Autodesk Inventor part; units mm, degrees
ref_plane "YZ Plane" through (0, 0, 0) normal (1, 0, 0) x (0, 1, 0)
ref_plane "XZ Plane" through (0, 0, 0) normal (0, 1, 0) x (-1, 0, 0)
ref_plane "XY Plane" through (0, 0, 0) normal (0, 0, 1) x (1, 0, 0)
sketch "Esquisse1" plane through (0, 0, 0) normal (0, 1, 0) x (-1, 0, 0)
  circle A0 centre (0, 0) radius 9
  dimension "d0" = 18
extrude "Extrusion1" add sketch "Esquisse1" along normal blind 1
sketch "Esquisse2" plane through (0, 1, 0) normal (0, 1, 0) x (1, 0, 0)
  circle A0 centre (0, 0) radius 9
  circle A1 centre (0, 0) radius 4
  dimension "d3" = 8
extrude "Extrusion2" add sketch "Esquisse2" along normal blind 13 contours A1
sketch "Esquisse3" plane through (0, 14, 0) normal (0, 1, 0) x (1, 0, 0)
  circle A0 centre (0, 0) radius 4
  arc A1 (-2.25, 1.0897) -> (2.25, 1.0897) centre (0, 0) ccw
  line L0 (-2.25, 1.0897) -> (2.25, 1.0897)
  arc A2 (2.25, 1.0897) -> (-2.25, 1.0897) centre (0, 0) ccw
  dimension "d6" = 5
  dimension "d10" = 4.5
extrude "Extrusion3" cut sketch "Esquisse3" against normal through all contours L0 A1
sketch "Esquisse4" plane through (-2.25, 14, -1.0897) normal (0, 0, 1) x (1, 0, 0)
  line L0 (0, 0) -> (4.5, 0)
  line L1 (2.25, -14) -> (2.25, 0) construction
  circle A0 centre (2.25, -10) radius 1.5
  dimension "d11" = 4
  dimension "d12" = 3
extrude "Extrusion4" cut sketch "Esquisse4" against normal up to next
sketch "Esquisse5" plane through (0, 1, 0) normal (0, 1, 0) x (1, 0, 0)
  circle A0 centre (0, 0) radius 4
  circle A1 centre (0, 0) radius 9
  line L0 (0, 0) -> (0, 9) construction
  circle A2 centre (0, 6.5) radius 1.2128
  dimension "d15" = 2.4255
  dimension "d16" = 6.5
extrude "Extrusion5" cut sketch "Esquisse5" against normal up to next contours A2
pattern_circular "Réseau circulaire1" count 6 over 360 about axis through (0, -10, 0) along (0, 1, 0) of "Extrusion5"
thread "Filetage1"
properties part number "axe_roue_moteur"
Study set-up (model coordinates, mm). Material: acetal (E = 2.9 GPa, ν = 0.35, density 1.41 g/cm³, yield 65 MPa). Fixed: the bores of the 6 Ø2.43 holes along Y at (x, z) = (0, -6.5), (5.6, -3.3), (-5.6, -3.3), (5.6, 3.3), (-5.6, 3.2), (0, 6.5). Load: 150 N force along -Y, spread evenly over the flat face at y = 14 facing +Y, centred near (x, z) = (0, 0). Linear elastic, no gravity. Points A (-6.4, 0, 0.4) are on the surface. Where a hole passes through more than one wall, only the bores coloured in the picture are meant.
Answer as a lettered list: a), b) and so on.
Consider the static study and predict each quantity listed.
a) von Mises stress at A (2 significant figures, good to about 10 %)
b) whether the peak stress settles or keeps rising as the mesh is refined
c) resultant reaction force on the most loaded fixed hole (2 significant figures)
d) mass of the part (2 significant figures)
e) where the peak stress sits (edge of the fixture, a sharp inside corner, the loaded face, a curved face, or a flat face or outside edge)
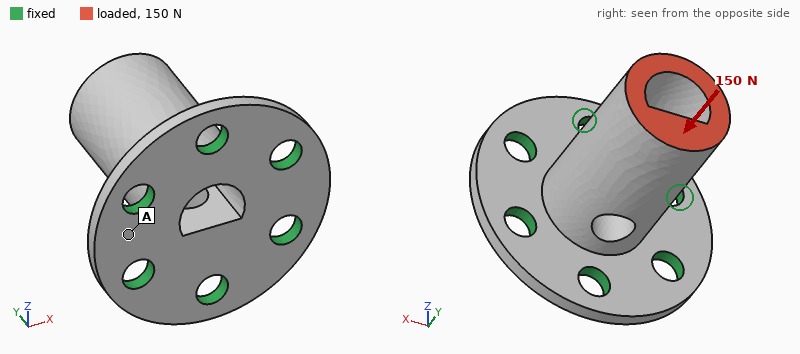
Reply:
a) 6.3 MPa
b) keeps rising
c) 30 N
d) 0.91 g
e) edge of the fixture
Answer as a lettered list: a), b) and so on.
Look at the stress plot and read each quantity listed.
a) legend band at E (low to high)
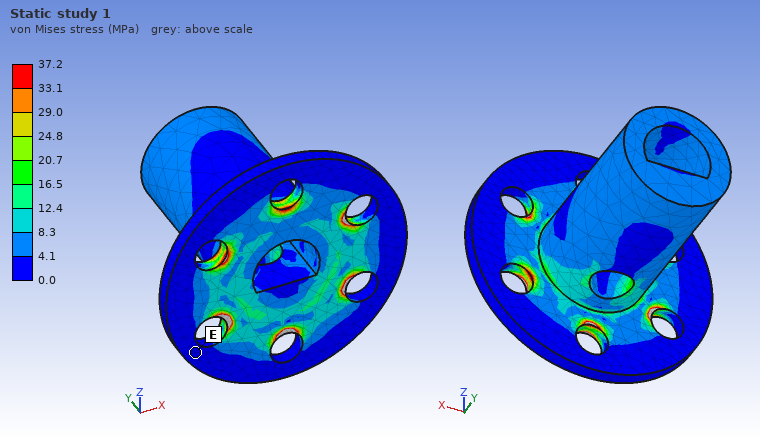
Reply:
a) 0.0 to 4.1 MPa
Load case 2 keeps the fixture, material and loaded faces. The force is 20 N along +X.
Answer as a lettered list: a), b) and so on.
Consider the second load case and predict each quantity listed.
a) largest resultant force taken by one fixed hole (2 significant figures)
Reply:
a) 17 N
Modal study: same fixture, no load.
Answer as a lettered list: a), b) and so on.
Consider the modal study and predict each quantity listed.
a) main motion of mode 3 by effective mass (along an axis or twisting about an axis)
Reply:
a) along Y
